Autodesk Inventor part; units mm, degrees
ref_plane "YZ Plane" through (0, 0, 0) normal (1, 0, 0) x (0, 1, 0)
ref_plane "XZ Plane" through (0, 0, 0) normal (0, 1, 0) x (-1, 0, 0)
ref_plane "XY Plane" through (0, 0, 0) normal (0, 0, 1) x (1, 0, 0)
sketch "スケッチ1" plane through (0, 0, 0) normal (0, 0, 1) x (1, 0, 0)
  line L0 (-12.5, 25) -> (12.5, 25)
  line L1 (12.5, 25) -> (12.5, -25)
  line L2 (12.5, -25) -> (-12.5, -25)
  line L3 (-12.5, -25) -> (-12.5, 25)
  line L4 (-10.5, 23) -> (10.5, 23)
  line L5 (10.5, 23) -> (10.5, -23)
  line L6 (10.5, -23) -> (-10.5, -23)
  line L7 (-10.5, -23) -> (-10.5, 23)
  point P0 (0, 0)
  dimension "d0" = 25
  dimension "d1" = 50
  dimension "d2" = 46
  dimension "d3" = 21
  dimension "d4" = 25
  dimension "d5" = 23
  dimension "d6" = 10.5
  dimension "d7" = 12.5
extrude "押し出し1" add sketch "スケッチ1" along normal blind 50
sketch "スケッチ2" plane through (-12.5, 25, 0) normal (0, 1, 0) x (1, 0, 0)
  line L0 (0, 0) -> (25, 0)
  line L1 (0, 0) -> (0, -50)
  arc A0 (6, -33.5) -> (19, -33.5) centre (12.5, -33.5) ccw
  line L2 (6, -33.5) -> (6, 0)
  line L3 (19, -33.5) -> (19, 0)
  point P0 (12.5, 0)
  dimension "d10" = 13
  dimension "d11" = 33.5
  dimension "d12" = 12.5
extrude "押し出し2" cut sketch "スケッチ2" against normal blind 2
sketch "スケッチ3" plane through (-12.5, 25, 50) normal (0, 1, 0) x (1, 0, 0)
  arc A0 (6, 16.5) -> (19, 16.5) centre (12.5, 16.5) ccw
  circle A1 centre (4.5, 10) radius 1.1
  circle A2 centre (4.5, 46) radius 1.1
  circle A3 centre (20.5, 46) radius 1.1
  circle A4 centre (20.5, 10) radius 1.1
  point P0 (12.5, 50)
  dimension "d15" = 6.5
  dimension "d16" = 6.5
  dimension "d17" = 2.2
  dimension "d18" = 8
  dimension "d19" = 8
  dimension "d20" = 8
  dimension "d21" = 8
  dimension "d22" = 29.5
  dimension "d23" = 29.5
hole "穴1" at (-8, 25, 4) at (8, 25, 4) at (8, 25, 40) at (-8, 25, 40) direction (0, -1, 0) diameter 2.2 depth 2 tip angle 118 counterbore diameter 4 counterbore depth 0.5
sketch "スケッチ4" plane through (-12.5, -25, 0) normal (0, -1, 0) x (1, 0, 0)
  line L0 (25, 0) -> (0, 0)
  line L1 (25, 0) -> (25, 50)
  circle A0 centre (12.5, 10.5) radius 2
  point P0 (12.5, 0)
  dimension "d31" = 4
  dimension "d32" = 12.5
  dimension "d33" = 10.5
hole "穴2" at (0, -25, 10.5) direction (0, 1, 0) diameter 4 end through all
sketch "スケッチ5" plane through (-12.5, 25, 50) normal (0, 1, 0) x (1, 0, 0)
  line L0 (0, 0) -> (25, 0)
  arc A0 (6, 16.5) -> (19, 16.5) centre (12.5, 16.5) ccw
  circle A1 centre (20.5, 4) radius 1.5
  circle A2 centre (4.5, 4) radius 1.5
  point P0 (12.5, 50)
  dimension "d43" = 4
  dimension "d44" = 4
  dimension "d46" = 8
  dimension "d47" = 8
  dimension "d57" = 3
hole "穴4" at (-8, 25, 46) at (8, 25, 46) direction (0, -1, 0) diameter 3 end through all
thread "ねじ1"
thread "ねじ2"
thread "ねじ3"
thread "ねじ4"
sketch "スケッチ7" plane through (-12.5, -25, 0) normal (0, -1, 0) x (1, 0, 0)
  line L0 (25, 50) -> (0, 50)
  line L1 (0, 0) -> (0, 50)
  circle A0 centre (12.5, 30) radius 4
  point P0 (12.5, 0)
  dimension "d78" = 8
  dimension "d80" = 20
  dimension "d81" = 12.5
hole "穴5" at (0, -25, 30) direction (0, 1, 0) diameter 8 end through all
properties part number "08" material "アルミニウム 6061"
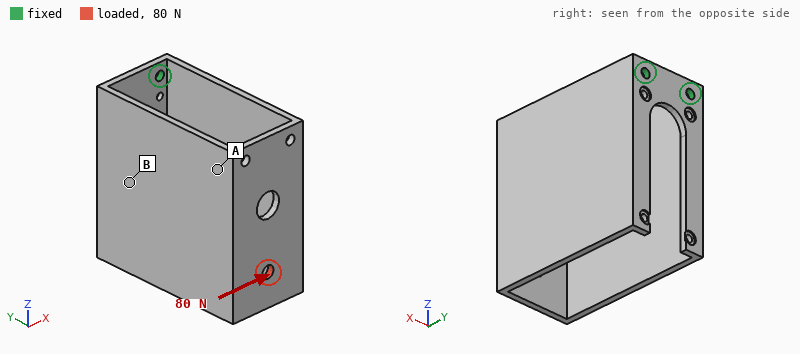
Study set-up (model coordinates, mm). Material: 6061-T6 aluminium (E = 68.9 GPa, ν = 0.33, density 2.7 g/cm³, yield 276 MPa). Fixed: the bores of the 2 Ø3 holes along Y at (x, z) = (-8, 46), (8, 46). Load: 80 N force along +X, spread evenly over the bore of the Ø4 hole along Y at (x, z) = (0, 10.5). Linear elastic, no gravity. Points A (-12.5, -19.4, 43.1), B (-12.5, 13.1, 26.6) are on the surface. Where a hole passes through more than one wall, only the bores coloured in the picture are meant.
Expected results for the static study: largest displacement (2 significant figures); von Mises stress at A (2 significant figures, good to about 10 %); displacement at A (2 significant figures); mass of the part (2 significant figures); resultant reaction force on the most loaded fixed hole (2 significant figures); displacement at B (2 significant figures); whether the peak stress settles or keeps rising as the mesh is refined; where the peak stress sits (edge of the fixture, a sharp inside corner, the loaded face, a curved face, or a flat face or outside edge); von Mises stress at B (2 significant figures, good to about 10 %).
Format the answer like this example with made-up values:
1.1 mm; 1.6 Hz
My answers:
0.42 mm; 25 MPa; 0.33 mm; 35 g; 190 N; 0.10 mm; keeps rising; edge of the fixture; 7.9 MPa
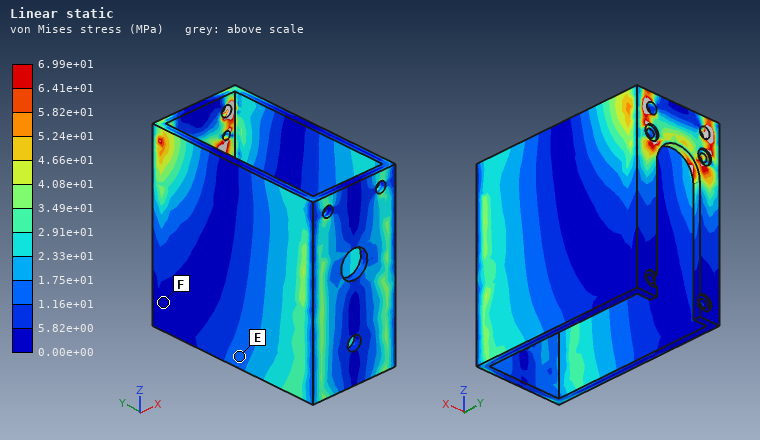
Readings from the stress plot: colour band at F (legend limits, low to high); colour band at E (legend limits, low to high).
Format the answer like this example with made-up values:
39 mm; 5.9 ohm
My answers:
0.00e+00 to 5.82e+00 MPa; 1.16e+01 to 1.75e+01 MPa
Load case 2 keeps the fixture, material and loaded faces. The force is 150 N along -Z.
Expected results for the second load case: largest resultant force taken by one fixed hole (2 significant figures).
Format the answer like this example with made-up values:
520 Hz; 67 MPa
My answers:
76 N
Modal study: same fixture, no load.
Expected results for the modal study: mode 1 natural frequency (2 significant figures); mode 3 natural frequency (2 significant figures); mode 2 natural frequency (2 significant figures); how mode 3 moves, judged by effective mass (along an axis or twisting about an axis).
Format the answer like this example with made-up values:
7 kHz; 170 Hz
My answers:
560 Hz; 1100 Hz; 570 Hz; twisting about Y
